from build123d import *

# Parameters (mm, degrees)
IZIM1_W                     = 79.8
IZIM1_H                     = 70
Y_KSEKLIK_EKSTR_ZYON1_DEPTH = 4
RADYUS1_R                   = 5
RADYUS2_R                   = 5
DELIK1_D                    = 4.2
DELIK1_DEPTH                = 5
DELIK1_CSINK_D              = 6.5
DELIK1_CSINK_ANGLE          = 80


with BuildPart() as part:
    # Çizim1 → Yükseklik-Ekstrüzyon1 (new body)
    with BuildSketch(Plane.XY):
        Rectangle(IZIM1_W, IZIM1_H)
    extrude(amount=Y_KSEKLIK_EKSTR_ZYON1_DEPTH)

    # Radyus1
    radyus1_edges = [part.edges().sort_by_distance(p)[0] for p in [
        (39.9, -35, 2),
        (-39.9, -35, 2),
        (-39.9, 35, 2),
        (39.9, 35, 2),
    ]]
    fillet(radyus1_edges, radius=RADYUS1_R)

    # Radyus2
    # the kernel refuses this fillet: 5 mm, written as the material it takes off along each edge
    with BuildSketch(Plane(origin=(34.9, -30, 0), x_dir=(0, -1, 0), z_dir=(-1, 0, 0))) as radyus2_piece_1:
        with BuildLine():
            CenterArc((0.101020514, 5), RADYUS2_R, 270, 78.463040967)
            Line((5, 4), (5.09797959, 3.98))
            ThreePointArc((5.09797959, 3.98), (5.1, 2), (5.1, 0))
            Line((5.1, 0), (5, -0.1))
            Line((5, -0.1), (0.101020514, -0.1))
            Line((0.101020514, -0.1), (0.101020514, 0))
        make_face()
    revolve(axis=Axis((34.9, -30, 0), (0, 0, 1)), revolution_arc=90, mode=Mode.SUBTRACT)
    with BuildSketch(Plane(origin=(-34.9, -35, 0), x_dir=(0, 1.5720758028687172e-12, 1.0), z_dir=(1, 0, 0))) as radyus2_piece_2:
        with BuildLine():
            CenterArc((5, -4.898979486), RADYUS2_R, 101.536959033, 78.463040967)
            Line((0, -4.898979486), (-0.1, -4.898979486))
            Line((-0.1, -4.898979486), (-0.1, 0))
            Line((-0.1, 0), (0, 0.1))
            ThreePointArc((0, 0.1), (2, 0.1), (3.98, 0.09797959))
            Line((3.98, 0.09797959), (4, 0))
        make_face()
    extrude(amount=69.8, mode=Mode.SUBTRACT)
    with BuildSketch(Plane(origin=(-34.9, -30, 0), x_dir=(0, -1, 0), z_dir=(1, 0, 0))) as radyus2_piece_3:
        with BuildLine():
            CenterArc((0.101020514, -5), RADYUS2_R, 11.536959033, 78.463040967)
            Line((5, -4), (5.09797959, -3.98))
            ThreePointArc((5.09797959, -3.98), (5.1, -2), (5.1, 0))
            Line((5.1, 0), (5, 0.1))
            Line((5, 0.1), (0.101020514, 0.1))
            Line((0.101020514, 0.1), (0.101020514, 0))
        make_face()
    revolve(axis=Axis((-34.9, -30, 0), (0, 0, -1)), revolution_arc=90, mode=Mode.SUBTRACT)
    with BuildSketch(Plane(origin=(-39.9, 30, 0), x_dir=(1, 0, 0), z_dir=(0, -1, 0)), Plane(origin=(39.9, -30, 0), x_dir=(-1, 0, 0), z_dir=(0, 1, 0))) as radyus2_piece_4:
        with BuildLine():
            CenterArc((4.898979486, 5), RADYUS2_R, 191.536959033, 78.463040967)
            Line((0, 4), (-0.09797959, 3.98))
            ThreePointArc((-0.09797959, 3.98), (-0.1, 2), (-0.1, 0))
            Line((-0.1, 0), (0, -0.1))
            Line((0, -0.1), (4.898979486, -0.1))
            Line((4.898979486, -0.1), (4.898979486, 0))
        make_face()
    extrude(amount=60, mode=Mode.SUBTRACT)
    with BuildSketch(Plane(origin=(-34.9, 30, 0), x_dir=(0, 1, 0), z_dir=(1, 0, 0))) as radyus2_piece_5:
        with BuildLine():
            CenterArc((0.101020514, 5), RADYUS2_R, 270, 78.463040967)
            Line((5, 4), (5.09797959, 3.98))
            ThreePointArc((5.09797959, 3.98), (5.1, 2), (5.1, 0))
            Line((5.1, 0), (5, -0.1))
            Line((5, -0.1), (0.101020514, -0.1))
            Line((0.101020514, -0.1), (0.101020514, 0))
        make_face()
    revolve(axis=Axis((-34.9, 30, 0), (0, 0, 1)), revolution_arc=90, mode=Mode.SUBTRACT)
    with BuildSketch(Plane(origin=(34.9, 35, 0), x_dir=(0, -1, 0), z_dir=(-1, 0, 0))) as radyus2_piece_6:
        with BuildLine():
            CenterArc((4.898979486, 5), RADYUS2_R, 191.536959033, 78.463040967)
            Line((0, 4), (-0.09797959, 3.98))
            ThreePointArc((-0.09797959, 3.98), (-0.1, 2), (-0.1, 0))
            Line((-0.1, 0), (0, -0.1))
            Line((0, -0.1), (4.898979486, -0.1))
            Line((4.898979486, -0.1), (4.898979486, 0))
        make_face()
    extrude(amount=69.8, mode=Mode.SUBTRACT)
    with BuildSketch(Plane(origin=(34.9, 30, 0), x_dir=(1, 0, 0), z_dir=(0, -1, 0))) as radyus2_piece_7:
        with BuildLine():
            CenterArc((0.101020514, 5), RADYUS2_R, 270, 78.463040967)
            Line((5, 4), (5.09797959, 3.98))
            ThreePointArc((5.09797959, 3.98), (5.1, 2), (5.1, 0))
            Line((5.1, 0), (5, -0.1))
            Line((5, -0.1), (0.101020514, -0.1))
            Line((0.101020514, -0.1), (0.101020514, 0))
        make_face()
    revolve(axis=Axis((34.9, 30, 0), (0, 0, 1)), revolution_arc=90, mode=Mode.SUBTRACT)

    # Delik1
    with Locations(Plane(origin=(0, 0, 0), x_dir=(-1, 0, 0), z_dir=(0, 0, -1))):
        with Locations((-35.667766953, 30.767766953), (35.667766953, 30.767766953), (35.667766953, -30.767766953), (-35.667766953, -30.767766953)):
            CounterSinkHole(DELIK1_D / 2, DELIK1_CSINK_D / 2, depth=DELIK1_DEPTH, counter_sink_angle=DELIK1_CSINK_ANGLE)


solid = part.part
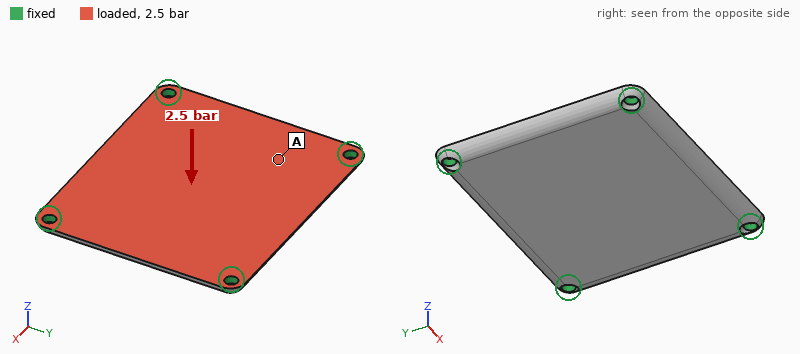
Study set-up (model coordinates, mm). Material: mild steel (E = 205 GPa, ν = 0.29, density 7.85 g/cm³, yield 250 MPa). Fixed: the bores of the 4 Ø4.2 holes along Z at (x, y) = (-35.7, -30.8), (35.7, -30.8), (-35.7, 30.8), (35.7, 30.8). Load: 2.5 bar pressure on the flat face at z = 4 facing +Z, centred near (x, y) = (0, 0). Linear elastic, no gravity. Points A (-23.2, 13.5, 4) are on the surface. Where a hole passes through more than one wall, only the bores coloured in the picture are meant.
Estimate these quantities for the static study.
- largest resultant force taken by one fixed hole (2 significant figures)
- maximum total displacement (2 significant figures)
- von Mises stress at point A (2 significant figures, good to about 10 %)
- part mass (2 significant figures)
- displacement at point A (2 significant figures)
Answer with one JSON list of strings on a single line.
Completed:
["440 N", "44 µm", "15 MPa", "160 g", "26 µm"]
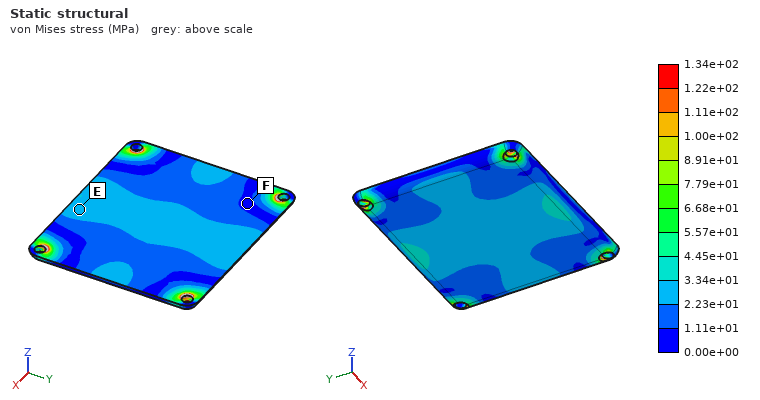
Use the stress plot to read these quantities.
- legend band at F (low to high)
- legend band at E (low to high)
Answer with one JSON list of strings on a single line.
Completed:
["0.00e+00 to 1.11e+01 MPa", "2.23e+01 to 3.34e+01 MPa"]
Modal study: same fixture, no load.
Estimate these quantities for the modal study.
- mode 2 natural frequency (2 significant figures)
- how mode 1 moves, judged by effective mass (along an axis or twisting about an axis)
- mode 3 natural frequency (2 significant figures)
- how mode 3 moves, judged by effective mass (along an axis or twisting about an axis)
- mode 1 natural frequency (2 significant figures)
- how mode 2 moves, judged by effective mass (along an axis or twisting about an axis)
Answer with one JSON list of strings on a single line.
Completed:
["4400 Hz", "along Z", "5100 Hz", "twisting about Y", "2600 Hz", "twisting about X"]
